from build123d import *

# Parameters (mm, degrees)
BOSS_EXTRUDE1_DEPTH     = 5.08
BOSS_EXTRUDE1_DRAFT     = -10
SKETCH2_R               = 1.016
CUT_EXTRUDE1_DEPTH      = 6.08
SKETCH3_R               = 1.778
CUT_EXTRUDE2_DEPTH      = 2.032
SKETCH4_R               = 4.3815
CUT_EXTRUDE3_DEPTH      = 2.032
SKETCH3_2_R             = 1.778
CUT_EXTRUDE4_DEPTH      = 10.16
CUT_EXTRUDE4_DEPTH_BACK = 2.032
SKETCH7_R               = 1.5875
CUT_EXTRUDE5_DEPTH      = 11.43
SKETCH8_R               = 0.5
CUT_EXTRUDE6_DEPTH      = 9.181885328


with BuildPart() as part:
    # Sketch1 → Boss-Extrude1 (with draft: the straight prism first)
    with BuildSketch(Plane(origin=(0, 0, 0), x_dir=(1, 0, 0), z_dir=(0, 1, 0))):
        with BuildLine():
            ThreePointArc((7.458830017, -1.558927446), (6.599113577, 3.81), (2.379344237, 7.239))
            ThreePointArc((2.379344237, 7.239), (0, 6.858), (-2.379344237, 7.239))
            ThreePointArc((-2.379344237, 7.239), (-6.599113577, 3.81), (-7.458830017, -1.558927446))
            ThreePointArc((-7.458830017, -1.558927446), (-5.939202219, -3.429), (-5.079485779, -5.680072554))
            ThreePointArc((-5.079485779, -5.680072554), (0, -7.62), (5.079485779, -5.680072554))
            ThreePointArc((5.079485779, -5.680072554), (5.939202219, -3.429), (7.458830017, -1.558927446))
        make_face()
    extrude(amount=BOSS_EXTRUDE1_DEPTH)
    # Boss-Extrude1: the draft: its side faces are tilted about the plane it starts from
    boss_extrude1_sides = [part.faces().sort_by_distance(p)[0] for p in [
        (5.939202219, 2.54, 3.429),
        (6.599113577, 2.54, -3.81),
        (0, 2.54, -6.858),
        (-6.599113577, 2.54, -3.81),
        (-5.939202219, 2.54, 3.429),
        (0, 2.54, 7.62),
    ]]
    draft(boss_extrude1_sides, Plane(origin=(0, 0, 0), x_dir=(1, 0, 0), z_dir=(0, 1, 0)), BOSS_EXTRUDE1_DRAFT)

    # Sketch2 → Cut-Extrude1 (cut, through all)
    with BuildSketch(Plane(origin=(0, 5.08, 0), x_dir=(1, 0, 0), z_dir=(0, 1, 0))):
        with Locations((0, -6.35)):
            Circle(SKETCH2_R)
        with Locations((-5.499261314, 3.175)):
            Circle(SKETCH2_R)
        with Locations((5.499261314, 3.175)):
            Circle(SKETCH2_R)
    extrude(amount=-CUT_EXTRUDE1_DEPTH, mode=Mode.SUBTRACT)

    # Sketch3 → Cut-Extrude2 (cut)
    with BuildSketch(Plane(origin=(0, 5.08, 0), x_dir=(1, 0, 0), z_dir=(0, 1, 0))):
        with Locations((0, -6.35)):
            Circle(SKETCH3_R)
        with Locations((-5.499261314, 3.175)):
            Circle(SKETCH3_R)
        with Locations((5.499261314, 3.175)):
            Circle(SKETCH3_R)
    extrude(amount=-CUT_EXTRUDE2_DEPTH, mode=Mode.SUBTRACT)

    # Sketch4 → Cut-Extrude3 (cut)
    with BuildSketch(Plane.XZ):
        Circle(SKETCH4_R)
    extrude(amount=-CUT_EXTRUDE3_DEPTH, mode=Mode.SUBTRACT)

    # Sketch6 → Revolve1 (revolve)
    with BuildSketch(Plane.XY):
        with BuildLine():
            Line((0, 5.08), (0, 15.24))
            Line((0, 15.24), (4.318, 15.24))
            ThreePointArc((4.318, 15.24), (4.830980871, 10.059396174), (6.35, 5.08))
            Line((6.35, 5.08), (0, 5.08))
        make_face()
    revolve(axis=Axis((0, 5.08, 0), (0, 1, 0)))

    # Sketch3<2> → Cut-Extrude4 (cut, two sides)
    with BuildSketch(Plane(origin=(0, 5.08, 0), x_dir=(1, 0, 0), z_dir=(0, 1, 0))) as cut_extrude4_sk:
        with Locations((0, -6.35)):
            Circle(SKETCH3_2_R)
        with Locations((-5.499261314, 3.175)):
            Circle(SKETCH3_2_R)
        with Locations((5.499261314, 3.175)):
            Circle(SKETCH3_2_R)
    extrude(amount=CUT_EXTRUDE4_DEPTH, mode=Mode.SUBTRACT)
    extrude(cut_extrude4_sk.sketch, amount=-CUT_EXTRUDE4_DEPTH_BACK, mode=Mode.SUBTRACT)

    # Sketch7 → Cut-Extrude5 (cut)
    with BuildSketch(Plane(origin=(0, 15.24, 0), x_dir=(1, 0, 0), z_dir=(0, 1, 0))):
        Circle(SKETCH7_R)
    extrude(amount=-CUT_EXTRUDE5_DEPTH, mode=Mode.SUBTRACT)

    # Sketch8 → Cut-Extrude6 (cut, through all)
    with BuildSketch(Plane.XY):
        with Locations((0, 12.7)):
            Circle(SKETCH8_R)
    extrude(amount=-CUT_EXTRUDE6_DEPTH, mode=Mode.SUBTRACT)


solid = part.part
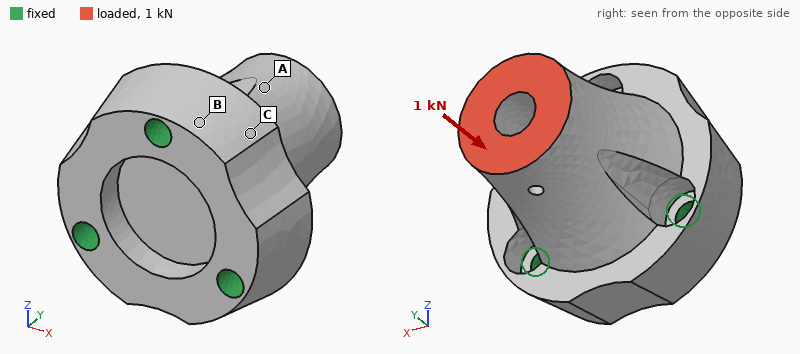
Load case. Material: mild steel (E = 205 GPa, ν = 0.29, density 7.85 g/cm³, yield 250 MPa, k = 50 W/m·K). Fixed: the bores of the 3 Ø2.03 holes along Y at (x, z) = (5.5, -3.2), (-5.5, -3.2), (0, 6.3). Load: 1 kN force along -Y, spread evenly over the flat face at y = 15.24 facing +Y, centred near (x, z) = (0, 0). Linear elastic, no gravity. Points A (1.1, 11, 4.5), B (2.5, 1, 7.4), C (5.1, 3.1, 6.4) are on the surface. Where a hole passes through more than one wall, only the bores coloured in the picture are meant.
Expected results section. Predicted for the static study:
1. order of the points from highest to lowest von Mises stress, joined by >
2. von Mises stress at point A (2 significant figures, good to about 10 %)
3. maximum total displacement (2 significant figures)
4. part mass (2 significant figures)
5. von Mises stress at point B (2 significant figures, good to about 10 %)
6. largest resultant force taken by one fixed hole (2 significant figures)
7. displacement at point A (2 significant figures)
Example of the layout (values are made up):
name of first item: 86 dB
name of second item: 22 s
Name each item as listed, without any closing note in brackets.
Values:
order of the points from highest to lowest von Mises stress, joined by >: A > B > C
von Mises stress at point A: 16 MPa
maximum total displacement: 1.5 µm
part mass: 12 g
von Mises stress at point B: 11 MPa
largest resultant force taken by one fixed hole: 350 N
displacement at point A: 1.0 µm
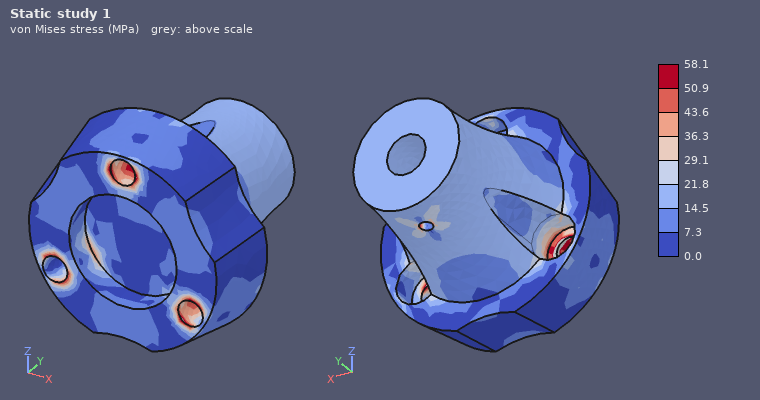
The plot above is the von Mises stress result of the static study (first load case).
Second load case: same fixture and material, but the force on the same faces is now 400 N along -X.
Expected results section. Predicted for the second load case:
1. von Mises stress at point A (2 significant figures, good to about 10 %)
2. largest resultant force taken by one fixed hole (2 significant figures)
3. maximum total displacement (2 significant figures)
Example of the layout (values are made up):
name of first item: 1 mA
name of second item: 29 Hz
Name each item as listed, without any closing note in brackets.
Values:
von Mises stress at point A: 15 MPa
largest resultant force taken by one fixed hole: 480 N
maximum total displacement: 5.1 µm
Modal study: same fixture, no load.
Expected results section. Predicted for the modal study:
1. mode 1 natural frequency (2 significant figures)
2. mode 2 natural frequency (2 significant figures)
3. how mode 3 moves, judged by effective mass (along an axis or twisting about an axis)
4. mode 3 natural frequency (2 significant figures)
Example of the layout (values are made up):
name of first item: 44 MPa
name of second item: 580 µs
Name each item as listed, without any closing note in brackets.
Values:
mode 1 natural frequency: 33 kHz
mode 2 natural frequency: 33 kHz
how mode 3 moves, judged by effective mass: along Y
mode 3 natural frequency: 61 kHz
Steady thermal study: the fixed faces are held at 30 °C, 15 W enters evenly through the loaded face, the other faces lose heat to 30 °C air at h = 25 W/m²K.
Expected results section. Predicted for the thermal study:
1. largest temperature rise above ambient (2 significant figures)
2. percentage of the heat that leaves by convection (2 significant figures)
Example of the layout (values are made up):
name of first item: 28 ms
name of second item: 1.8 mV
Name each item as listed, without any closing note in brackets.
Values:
largest temperature rise above ambient: 64 K
percentage of the heat that leaves by convection: 3.5 %
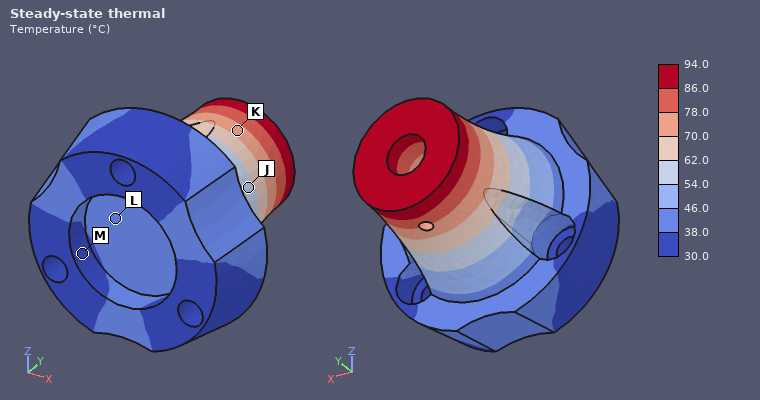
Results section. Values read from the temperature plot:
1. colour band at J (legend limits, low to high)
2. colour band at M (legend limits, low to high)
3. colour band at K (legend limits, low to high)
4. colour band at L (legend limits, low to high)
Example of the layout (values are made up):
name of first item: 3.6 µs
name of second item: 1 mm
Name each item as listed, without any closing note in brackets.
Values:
colour band at J: 54.0 to 62.0 °C
colour band at M: 30.0 to 38.0 °C
colour band at K: 70.0 to 78.0 °C
colour band at L: 38.0 to 46.0 °C
